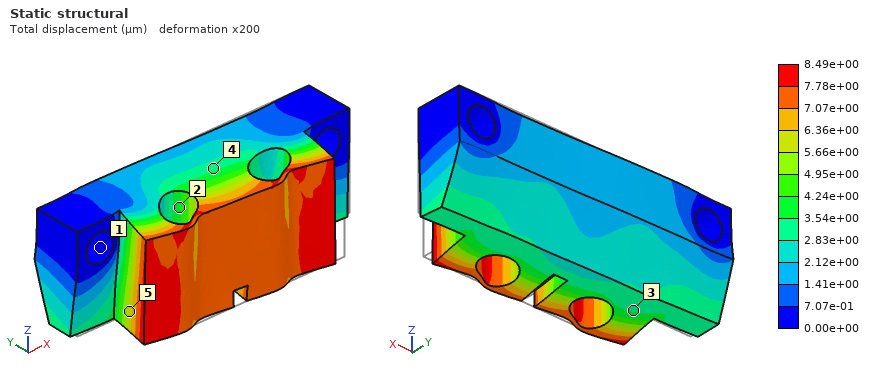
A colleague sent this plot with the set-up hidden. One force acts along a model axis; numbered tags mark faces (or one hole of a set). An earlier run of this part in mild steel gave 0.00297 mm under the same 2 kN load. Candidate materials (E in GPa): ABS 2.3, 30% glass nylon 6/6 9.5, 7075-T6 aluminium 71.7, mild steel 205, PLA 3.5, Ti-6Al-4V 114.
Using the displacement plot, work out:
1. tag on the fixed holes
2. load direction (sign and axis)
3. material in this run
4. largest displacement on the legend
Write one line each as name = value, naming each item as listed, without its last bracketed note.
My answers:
tag on the fixed holes = 1
load direction = -X
material in this run = 7075-T6 aluminium
largest displacement on the legend = 8.49e+00 µm
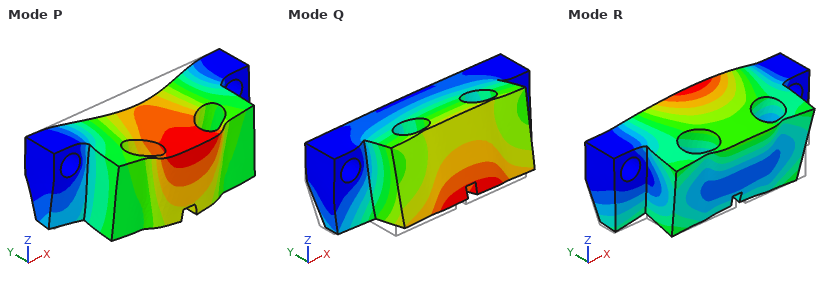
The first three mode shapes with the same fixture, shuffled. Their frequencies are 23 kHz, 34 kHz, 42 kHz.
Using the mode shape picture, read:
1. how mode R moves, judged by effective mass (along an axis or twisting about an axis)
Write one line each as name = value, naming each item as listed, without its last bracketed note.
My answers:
how mode R moves, judged by effective mass = along Z
